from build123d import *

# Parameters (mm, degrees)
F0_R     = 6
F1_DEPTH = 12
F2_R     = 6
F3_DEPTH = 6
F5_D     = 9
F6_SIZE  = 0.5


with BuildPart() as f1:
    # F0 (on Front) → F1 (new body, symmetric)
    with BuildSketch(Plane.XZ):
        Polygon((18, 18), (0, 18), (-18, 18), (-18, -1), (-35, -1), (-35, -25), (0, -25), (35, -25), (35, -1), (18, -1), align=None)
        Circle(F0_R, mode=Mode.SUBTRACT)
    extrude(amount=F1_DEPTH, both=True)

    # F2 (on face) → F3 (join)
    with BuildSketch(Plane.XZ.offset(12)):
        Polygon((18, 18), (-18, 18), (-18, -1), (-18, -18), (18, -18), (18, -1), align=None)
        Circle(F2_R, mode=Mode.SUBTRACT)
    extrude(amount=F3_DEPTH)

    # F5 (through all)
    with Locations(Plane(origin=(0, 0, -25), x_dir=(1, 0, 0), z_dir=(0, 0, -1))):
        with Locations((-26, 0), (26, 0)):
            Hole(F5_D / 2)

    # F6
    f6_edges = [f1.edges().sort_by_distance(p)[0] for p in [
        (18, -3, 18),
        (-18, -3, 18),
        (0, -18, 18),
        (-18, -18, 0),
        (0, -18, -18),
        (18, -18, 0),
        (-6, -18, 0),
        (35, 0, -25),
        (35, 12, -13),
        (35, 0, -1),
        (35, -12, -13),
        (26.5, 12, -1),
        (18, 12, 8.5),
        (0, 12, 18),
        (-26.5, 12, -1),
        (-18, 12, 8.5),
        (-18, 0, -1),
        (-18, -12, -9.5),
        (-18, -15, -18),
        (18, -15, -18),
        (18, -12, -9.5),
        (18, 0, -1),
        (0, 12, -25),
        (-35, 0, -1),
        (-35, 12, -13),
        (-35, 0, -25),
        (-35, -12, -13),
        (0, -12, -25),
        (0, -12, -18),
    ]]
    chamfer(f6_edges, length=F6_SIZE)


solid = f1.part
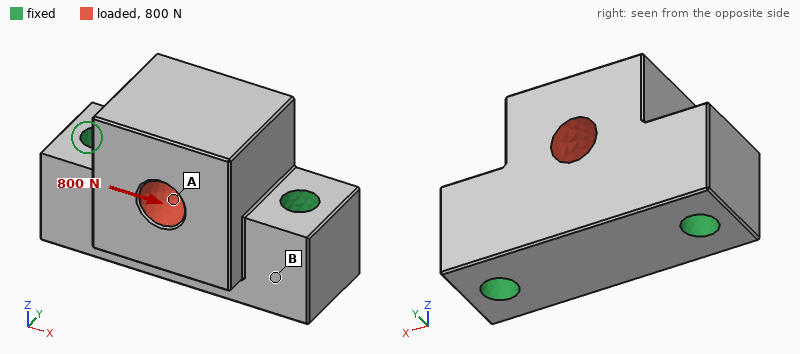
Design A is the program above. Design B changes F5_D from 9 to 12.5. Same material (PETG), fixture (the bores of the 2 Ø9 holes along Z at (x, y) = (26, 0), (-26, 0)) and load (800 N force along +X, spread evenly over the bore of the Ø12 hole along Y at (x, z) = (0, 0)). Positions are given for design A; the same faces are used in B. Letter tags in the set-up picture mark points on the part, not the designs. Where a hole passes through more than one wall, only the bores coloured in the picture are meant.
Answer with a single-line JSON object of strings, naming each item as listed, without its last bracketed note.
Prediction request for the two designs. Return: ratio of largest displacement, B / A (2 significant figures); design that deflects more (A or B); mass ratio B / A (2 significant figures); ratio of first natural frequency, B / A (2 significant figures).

{"ratio of largest displacement, B / A": "0.90", "design that deflects more": "A", "mass ratio B / A": "0.95", "ratio of first natural frequency, B / A": "1.1"}
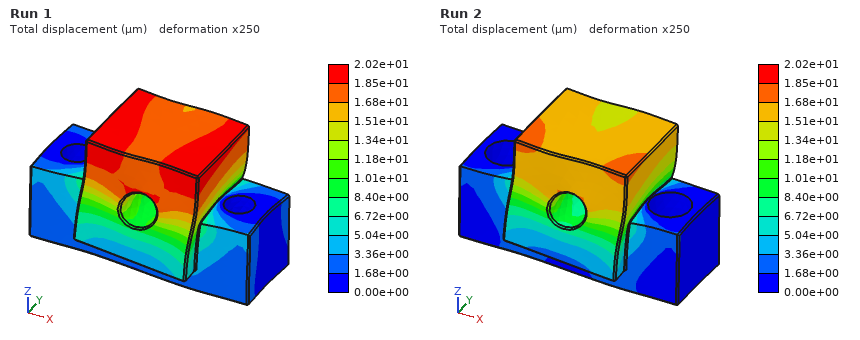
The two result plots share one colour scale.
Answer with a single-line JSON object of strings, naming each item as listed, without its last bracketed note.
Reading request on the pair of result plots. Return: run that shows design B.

{"run that shows design B": "Run 2"}
